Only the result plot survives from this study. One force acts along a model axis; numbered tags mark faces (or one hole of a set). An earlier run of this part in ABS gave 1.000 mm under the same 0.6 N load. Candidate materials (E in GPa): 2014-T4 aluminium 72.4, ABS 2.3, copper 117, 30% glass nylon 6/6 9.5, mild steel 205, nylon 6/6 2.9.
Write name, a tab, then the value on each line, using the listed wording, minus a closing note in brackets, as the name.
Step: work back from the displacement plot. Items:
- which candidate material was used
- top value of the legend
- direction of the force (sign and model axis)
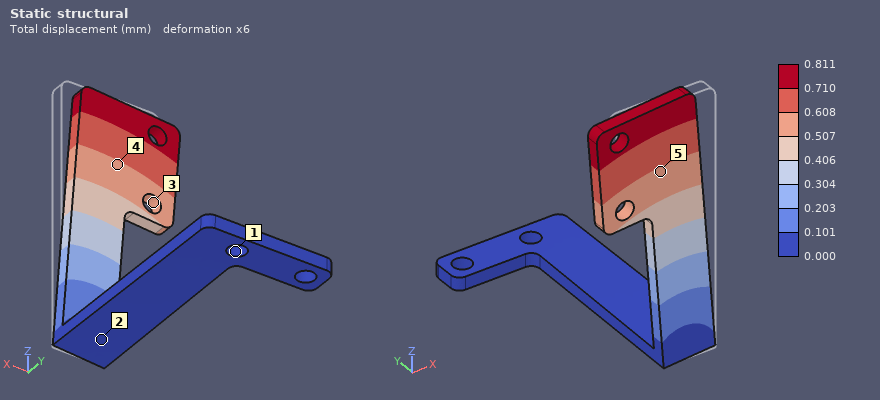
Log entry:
which candidate material was used	nylon 6/6
top value of the legend	0.811 mm
direction of the force	-X
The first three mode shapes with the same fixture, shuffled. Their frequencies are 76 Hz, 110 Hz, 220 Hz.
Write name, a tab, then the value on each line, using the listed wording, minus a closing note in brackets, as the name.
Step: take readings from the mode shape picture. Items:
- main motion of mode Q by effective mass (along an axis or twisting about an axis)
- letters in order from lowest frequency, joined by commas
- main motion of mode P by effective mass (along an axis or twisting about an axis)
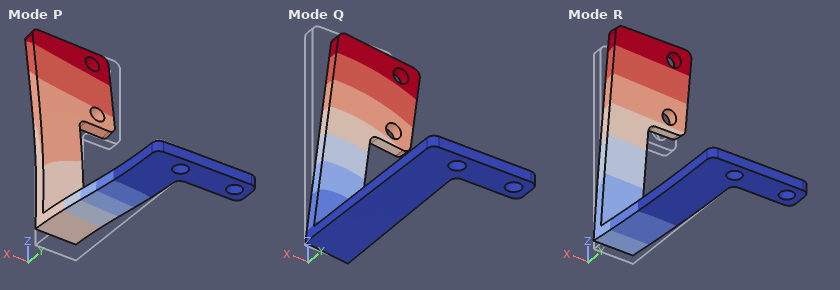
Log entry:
main motion of mode Q by effective mass	along X
letters in order from lowest frequency, joined by commas	R, Q, P
main motion of mode P by effective mass	along Z
